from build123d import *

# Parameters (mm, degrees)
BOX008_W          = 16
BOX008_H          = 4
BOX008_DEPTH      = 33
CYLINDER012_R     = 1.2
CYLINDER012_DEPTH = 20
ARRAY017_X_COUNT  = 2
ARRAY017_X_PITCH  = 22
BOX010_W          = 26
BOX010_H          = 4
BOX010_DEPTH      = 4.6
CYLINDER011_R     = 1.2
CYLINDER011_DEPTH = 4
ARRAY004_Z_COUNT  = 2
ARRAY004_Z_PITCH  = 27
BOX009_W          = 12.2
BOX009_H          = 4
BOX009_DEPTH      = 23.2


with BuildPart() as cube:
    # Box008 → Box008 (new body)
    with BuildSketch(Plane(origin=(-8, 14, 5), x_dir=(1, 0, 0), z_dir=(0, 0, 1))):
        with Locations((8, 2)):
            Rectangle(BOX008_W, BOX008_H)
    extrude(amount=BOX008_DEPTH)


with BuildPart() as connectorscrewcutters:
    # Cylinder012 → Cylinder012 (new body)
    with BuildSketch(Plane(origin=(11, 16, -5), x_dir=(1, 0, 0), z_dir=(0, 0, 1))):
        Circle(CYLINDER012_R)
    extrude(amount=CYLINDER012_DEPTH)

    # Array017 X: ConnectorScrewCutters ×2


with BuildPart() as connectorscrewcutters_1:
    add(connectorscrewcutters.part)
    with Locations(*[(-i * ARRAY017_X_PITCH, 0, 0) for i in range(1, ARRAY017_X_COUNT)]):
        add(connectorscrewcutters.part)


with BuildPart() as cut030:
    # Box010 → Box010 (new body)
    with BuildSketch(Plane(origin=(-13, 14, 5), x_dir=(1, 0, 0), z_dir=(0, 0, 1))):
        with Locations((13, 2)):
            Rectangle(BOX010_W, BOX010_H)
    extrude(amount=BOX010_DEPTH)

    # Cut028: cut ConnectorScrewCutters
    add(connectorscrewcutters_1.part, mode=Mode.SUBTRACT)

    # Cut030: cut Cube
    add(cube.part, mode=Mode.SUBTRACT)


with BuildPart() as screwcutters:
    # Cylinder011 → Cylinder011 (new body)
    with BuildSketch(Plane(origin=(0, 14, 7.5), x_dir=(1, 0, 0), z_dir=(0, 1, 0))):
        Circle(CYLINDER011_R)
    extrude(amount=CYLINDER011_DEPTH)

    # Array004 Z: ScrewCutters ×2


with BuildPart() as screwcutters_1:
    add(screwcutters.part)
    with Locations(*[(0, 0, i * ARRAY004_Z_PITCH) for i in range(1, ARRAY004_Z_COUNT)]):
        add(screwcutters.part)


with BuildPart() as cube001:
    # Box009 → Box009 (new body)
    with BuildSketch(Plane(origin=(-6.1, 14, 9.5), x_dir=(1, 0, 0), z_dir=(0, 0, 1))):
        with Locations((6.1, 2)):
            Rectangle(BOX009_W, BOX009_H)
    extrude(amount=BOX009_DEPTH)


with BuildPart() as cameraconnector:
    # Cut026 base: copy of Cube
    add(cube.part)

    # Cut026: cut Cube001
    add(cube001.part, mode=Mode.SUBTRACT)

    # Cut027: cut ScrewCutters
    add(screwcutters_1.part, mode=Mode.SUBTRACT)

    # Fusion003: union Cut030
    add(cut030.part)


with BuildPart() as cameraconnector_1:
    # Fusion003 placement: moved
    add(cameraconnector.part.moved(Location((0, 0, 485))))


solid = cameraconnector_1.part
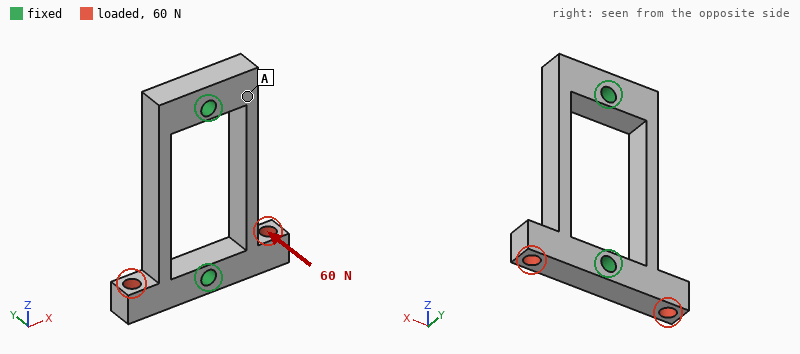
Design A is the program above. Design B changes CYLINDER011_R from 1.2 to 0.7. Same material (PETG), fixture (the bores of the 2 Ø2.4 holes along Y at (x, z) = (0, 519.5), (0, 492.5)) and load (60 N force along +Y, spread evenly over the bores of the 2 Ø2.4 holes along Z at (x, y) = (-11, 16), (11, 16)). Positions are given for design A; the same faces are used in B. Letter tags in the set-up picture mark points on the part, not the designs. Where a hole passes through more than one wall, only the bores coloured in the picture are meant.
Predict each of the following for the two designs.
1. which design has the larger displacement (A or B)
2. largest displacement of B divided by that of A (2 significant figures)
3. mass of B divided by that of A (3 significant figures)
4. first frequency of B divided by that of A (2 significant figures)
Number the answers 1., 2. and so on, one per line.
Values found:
1. B
2. 1.1
3. 1.02
4. 0.98
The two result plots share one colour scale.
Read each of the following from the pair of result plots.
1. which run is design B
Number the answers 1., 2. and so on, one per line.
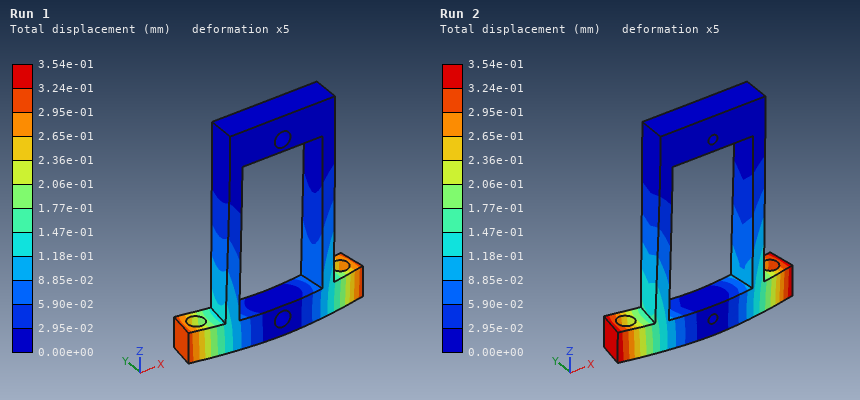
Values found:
1. Run 2
